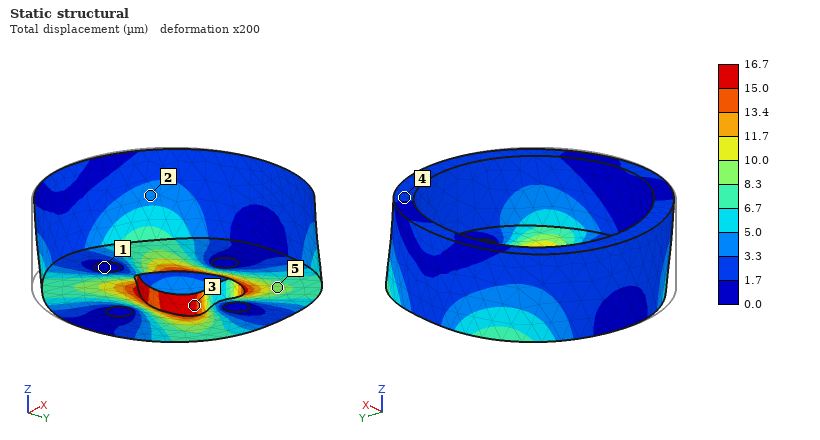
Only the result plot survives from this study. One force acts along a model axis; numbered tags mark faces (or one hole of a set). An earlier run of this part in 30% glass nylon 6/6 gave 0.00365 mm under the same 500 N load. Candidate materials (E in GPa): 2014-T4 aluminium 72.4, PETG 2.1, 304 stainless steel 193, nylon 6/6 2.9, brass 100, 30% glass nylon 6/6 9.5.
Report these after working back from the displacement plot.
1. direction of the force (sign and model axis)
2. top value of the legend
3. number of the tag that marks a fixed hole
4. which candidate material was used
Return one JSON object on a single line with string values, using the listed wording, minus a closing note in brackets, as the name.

{"direction of the force": "+Y", "top value of the legend": "16.7 µm", "number of the tag that marks a fixed hole": "1", "which candidate material was used": "PETG"}
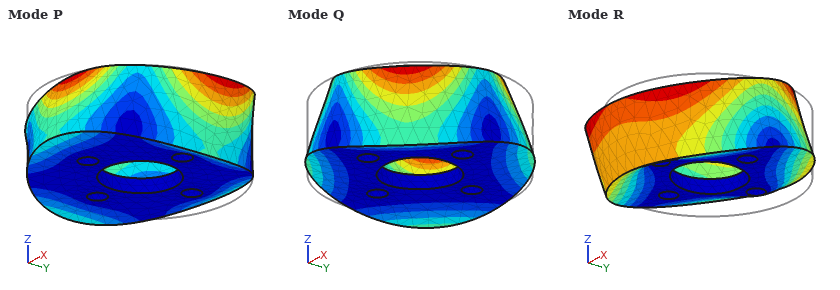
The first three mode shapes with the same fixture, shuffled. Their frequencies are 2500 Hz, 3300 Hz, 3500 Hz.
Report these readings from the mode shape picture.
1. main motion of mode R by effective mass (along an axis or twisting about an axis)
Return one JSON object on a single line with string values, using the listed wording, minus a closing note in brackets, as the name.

{"main motion of mode R by effective mass": "along Y"}
